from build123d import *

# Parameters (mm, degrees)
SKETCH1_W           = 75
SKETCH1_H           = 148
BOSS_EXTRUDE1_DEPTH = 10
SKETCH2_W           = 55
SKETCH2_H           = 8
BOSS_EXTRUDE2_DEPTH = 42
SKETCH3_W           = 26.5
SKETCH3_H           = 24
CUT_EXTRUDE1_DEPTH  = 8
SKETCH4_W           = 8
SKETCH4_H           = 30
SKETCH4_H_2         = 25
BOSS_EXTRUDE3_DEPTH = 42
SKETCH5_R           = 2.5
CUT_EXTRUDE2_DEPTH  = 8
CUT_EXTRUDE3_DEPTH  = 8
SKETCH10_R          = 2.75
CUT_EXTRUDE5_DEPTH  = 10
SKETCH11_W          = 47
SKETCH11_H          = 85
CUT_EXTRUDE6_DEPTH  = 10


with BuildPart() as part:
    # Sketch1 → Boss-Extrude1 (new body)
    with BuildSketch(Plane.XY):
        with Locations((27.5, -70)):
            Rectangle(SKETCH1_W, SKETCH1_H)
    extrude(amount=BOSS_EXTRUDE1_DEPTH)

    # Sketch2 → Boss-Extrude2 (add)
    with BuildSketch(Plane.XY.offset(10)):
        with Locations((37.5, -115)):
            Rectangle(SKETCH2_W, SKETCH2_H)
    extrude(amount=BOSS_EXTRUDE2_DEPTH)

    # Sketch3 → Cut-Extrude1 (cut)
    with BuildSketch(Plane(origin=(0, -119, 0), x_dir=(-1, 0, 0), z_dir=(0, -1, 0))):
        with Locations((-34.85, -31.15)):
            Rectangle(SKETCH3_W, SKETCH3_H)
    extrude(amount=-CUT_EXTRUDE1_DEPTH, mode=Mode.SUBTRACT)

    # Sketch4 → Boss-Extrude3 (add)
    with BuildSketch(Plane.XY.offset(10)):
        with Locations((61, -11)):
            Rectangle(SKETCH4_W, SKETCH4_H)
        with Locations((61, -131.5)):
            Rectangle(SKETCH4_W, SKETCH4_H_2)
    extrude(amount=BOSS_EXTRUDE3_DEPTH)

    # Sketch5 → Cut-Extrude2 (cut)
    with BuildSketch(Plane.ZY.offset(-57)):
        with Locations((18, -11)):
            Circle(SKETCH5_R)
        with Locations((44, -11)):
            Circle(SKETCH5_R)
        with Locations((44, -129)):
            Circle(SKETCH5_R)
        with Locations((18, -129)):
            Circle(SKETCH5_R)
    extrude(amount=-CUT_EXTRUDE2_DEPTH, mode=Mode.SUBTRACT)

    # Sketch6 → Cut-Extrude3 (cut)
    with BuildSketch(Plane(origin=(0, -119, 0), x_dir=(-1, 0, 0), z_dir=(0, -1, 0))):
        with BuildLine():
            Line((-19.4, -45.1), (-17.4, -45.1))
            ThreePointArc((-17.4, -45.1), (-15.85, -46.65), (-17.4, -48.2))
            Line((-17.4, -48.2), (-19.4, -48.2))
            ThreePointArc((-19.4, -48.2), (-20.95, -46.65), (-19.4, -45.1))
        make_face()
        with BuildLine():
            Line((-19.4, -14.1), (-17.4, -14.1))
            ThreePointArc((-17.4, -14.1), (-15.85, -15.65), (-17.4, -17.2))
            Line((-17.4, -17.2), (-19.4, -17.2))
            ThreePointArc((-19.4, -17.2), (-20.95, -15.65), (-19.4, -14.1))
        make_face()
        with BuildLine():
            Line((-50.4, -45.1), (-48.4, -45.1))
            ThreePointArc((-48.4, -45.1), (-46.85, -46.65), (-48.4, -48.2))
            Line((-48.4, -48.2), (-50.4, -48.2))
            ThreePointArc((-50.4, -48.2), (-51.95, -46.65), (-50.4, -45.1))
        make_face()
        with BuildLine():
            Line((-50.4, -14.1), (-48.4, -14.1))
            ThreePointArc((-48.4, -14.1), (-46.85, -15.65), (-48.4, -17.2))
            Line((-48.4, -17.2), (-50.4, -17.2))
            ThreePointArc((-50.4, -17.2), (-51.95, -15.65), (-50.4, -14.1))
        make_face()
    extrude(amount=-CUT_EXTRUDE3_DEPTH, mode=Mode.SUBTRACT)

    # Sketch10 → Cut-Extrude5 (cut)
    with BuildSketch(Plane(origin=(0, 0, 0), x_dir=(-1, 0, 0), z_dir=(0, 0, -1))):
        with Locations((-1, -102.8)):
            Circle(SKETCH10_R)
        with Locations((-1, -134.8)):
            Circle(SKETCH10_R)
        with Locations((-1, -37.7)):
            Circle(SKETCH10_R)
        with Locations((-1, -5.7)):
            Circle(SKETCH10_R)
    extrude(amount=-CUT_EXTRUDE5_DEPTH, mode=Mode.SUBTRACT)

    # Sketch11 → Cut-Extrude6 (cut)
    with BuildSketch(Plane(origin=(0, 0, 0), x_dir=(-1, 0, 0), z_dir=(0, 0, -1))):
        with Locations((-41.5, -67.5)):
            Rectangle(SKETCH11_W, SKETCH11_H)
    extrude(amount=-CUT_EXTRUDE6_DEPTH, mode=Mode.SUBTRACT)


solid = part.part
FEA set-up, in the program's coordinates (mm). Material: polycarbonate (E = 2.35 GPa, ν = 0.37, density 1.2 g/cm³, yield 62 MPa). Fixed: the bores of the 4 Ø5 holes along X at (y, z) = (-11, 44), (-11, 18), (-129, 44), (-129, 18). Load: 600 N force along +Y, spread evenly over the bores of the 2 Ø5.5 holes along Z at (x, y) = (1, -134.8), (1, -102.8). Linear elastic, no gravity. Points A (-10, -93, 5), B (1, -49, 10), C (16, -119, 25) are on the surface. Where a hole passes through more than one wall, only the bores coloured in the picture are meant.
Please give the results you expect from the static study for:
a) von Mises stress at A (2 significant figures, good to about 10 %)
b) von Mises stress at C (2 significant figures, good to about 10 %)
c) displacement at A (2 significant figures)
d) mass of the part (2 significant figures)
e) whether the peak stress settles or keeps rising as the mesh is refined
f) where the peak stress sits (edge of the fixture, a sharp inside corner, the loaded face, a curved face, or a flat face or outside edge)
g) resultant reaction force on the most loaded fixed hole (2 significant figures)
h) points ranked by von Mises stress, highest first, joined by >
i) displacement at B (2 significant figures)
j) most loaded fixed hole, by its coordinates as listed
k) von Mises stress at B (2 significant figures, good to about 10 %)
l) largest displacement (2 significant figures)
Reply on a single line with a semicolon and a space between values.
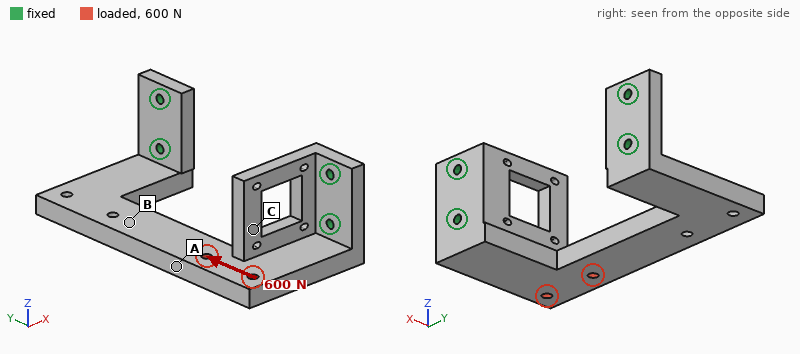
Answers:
6.3 MPa; 1.4 MPa; 0.57 mm; 120 g; keeps rising; edge of the fixture; 510 N; A > B > C; 0.56 mm; (-129, 18); 2.8 MPa; 0.69 mm
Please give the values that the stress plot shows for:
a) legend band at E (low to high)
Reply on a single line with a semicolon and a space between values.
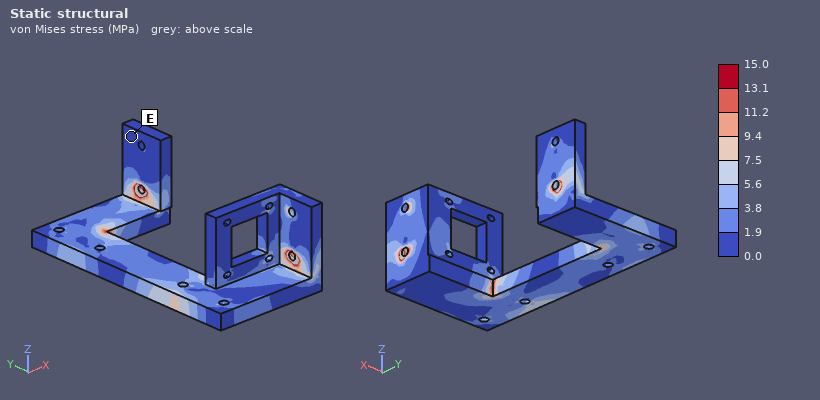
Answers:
0.0 to 1.9 MPa
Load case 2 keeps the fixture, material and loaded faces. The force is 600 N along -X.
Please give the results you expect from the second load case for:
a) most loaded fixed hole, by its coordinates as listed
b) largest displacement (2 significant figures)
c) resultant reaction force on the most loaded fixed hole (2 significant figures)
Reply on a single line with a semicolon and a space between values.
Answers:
(-129, 18); 0.50 mm; 680 N
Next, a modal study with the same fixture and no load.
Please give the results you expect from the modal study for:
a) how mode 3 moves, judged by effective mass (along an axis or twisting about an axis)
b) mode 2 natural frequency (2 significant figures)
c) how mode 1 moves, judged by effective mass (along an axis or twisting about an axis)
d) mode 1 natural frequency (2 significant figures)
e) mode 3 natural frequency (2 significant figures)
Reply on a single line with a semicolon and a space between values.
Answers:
along Y; 540 Hz; along Z; 290 Hz; 680 Hz
